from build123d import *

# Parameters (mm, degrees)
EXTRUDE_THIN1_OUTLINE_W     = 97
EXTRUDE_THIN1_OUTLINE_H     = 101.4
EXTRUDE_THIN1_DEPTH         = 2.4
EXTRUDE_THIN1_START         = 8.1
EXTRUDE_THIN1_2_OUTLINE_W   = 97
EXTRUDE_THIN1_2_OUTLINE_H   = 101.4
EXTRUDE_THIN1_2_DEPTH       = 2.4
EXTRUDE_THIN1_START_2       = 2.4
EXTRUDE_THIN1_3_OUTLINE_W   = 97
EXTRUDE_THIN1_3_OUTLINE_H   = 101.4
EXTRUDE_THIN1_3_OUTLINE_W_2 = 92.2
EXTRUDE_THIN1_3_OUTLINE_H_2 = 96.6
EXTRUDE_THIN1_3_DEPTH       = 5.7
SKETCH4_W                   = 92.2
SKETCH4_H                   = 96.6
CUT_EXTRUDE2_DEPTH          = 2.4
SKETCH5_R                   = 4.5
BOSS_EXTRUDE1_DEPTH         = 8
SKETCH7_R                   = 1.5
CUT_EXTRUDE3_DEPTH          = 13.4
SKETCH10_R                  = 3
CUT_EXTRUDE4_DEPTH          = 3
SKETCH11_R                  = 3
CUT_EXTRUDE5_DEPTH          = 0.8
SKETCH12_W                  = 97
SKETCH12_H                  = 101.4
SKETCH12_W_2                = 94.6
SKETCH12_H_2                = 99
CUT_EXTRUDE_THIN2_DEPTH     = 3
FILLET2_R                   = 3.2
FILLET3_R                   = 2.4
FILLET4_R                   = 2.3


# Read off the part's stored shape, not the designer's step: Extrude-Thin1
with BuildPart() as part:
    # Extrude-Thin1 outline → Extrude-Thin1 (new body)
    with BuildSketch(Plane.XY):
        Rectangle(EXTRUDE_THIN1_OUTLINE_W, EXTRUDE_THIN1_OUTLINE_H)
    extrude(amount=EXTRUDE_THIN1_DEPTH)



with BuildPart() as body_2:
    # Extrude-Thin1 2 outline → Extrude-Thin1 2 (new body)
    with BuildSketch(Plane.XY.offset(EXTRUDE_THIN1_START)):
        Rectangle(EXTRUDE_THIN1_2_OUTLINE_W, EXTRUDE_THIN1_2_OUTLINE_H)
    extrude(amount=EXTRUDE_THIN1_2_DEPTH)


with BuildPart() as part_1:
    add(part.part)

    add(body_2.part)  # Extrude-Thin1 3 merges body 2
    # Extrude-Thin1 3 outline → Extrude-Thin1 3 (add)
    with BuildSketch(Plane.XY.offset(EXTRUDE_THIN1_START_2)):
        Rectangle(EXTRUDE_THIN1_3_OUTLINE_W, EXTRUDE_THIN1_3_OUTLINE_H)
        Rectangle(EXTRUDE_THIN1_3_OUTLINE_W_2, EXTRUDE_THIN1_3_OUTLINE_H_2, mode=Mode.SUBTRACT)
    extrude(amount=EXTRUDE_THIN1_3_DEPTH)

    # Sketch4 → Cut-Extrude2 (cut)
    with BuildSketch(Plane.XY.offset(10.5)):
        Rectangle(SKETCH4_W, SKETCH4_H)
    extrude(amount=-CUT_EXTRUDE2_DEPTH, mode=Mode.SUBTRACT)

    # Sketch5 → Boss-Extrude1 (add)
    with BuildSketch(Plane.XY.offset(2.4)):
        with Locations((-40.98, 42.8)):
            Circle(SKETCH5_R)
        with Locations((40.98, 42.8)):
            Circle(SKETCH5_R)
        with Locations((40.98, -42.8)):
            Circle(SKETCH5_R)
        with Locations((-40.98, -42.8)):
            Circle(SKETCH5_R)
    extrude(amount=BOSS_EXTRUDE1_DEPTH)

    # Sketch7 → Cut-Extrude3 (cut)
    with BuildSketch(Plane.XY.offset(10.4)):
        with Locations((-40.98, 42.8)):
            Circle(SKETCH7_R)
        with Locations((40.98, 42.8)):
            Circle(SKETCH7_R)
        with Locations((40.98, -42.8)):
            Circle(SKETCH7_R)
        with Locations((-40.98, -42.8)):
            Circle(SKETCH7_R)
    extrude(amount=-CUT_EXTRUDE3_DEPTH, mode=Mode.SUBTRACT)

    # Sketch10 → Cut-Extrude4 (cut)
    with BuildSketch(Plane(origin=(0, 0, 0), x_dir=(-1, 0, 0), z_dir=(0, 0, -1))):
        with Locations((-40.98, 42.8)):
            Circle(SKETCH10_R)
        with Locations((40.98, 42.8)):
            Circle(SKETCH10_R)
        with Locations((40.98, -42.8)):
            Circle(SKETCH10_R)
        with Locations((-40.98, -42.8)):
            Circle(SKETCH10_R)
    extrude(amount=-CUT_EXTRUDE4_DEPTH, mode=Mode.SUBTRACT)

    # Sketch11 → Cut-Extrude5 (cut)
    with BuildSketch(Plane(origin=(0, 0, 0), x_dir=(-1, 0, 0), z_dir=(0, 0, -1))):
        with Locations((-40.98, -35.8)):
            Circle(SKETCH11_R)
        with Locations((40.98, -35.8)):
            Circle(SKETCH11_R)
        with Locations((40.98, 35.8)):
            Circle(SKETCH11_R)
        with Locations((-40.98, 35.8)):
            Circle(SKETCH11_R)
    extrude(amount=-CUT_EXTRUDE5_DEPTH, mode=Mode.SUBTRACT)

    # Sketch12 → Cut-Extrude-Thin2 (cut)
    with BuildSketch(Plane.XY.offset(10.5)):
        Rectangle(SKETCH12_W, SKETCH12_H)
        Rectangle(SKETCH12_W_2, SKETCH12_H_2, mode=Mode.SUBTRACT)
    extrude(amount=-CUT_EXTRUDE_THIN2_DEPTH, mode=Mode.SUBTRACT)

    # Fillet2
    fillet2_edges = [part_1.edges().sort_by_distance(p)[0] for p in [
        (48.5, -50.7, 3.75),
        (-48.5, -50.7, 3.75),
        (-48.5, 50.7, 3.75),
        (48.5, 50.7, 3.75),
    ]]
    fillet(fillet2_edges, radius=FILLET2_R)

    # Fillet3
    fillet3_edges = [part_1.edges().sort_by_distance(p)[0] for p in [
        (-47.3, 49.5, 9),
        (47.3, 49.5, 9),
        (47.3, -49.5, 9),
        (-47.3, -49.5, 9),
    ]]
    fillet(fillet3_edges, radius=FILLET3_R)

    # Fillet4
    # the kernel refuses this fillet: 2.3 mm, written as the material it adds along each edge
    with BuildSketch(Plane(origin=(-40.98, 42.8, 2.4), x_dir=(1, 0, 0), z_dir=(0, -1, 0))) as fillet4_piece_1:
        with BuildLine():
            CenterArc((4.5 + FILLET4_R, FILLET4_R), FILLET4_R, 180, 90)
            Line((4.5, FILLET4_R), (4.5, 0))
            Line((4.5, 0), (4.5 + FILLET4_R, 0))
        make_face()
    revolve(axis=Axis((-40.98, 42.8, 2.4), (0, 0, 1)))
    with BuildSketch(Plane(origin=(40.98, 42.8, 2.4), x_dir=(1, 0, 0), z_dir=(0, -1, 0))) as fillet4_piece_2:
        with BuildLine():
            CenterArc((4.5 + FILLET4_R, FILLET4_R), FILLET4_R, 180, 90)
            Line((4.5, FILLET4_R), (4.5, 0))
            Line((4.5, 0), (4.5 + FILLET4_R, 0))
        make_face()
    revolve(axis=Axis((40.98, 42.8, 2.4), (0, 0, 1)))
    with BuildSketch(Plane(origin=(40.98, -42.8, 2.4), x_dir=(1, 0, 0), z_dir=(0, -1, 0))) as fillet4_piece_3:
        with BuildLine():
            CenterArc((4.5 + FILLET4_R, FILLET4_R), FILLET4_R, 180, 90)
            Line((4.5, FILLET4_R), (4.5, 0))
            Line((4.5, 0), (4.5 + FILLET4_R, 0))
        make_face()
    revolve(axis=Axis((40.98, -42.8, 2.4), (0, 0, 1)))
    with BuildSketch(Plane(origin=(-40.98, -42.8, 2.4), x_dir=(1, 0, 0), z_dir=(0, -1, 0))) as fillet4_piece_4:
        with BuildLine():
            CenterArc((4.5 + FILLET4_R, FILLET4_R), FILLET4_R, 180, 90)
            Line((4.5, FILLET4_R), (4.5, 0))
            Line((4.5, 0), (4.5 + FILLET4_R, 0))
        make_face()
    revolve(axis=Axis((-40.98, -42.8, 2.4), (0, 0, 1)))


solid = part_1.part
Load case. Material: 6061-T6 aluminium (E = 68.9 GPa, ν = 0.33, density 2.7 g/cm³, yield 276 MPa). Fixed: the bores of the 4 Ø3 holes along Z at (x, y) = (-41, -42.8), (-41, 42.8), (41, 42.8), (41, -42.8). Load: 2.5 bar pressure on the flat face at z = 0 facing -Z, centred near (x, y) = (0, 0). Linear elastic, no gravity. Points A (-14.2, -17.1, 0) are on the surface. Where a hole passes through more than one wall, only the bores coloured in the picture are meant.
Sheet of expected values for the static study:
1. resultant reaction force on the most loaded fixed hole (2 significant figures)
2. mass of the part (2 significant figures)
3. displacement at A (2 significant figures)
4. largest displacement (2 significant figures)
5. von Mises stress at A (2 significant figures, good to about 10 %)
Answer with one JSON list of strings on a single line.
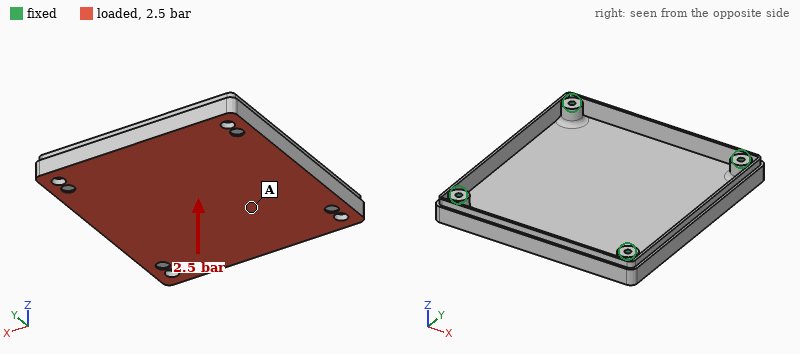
["1000 N", "84 g", "0.50 mm", "0.66 mm", "69 MPa"]
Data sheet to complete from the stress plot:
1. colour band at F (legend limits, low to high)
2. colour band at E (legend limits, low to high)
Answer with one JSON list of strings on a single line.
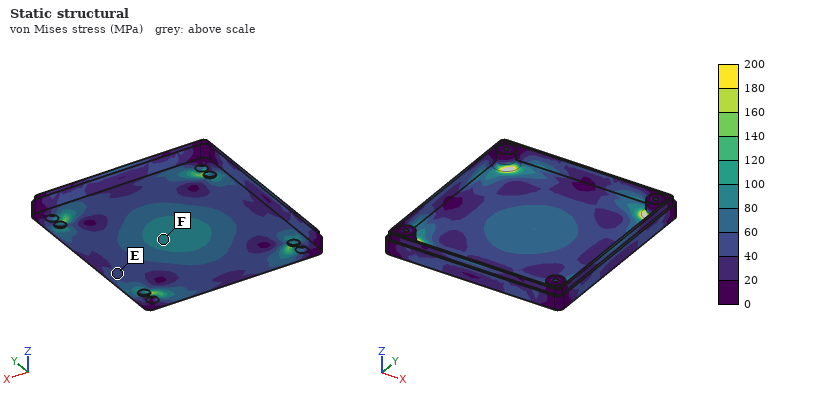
["80 to 100 MPa", "40 to 60 MPa"]
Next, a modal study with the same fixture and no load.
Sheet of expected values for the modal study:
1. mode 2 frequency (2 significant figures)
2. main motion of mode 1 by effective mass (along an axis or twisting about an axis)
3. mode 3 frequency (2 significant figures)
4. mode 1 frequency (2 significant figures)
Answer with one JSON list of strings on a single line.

["3100 Hz", "along Z", "3100 Hz", "1500 Hz"]
